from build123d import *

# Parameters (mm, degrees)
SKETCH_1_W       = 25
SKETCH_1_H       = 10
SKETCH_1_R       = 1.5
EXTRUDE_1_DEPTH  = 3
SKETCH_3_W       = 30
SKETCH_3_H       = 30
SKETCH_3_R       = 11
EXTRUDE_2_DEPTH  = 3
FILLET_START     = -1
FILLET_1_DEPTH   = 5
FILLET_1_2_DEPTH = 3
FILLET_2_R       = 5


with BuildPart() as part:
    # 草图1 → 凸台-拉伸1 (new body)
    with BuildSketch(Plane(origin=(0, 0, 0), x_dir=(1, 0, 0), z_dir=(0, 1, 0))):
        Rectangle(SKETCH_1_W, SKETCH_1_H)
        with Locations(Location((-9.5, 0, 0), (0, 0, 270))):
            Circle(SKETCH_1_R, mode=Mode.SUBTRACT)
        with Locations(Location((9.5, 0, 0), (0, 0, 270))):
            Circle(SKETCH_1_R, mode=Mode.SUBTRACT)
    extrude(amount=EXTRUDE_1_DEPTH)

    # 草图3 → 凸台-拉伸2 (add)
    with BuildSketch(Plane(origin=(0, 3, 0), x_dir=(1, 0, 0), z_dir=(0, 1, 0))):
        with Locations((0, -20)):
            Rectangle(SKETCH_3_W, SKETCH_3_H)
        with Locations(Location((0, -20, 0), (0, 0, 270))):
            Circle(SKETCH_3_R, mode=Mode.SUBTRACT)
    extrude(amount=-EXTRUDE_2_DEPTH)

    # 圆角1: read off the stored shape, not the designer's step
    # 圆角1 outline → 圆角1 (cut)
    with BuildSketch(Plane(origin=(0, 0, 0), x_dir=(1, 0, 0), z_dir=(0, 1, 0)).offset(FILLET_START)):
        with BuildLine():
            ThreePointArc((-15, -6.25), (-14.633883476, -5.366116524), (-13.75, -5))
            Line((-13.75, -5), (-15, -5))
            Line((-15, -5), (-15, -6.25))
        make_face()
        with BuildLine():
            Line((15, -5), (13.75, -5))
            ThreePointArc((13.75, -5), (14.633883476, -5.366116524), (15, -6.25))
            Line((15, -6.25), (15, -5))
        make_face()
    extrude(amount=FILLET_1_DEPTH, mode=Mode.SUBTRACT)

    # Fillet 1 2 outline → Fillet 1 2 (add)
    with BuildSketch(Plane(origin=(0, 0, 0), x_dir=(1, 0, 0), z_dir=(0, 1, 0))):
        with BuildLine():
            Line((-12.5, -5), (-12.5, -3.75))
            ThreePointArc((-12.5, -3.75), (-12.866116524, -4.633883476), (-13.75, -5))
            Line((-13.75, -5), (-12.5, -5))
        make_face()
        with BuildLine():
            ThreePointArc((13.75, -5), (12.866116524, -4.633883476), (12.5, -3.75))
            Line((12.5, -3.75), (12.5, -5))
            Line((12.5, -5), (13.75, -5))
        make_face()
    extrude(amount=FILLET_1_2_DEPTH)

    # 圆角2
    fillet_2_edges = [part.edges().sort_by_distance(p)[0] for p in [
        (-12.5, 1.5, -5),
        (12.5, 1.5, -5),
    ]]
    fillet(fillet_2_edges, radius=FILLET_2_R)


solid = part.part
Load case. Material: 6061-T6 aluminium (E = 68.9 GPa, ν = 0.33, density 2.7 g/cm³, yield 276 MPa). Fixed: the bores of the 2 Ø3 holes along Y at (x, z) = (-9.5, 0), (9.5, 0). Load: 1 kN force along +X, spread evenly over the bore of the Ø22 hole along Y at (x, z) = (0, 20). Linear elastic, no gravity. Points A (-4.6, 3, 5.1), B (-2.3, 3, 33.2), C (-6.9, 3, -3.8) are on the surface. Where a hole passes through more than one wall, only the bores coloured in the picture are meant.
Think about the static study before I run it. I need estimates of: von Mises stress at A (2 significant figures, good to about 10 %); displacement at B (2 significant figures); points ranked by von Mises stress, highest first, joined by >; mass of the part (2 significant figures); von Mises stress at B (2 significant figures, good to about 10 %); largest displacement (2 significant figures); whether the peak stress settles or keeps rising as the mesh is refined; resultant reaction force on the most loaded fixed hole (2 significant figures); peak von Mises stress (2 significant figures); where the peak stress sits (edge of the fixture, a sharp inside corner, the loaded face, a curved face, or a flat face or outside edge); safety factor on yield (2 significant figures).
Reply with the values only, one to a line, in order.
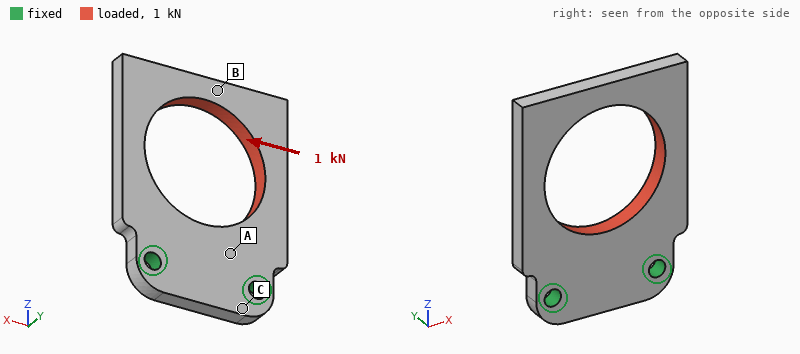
55 MPa
0.13 mm
A > B > C
6.0 g
29 MPa
0.14 mm
settles
1.1 kN
210 MPa
a curved face
1.3
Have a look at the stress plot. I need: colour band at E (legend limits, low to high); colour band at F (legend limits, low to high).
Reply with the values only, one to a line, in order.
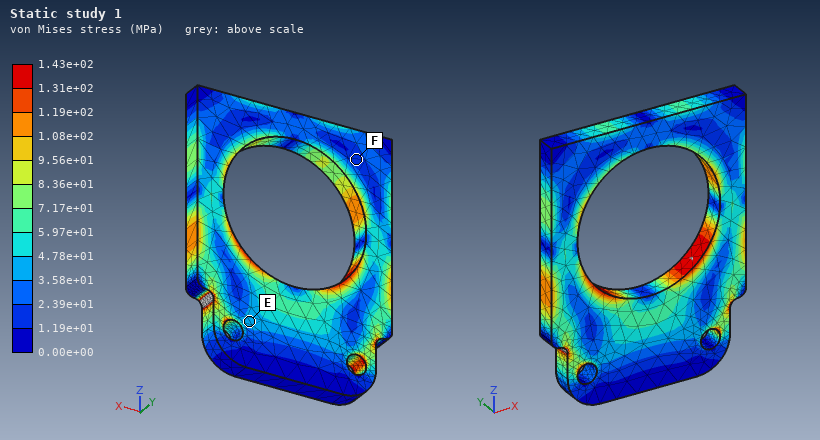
3.58e+01 to 4.78e+01 MPa
1.19e+01 to 2.39e+01 MPa
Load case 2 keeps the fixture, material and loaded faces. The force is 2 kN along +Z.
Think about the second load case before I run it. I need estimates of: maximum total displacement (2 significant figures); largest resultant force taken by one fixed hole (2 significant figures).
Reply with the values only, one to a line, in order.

56 µm
1.0 kN
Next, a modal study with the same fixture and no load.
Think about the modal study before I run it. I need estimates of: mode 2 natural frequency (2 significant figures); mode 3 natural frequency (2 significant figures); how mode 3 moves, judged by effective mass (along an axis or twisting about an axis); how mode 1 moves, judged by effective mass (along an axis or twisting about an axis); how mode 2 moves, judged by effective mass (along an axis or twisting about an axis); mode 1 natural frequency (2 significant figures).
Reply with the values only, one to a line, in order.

4100 Hz
7200 Hz
along X
along Y
twisting about Z
1800 Hz
